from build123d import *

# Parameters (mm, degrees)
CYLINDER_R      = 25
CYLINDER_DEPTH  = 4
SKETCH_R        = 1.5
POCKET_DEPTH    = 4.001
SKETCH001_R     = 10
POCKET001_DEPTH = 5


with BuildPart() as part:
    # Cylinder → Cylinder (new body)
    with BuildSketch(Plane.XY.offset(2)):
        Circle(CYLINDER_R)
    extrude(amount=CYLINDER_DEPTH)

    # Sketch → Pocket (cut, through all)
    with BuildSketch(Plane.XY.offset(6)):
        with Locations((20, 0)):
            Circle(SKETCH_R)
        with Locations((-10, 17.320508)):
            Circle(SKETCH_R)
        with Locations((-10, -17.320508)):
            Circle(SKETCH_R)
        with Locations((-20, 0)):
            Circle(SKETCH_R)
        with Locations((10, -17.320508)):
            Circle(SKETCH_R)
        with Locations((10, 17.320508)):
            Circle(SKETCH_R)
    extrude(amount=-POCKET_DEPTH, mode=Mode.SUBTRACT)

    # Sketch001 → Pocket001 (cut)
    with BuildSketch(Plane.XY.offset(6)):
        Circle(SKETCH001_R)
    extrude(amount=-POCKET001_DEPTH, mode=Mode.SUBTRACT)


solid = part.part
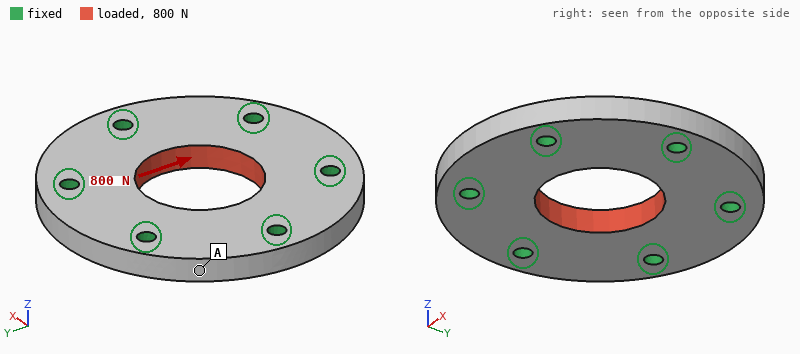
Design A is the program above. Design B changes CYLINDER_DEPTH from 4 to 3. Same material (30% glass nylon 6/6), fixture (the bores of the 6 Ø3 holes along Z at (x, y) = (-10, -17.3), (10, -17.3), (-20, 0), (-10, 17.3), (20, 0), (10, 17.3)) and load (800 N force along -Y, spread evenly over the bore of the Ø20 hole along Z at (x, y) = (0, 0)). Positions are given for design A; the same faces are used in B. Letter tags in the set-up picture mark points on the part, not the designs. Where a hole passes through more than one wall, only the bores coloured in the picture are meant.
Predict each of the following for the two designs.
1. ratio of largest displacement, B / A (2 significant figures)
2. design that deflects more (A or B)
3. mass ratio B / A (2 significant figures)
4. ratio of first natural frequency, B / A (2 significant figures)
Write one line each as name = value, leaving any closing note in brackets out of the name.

ratio of largest displacement, B / A = 1.3
design that deflects more = B
mass ratio B / A = 0.75
ratio of first natural frequency, B / A = 0.82
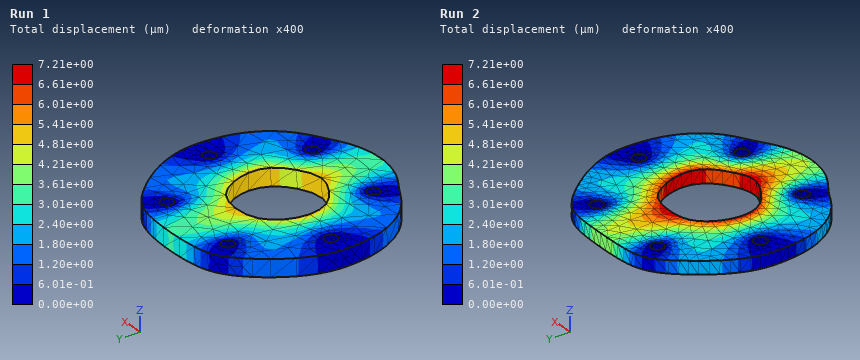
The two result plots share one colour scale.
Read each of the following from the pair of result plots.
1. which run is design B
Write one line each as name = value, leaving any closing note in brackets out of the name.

which run is design B = Run 2
